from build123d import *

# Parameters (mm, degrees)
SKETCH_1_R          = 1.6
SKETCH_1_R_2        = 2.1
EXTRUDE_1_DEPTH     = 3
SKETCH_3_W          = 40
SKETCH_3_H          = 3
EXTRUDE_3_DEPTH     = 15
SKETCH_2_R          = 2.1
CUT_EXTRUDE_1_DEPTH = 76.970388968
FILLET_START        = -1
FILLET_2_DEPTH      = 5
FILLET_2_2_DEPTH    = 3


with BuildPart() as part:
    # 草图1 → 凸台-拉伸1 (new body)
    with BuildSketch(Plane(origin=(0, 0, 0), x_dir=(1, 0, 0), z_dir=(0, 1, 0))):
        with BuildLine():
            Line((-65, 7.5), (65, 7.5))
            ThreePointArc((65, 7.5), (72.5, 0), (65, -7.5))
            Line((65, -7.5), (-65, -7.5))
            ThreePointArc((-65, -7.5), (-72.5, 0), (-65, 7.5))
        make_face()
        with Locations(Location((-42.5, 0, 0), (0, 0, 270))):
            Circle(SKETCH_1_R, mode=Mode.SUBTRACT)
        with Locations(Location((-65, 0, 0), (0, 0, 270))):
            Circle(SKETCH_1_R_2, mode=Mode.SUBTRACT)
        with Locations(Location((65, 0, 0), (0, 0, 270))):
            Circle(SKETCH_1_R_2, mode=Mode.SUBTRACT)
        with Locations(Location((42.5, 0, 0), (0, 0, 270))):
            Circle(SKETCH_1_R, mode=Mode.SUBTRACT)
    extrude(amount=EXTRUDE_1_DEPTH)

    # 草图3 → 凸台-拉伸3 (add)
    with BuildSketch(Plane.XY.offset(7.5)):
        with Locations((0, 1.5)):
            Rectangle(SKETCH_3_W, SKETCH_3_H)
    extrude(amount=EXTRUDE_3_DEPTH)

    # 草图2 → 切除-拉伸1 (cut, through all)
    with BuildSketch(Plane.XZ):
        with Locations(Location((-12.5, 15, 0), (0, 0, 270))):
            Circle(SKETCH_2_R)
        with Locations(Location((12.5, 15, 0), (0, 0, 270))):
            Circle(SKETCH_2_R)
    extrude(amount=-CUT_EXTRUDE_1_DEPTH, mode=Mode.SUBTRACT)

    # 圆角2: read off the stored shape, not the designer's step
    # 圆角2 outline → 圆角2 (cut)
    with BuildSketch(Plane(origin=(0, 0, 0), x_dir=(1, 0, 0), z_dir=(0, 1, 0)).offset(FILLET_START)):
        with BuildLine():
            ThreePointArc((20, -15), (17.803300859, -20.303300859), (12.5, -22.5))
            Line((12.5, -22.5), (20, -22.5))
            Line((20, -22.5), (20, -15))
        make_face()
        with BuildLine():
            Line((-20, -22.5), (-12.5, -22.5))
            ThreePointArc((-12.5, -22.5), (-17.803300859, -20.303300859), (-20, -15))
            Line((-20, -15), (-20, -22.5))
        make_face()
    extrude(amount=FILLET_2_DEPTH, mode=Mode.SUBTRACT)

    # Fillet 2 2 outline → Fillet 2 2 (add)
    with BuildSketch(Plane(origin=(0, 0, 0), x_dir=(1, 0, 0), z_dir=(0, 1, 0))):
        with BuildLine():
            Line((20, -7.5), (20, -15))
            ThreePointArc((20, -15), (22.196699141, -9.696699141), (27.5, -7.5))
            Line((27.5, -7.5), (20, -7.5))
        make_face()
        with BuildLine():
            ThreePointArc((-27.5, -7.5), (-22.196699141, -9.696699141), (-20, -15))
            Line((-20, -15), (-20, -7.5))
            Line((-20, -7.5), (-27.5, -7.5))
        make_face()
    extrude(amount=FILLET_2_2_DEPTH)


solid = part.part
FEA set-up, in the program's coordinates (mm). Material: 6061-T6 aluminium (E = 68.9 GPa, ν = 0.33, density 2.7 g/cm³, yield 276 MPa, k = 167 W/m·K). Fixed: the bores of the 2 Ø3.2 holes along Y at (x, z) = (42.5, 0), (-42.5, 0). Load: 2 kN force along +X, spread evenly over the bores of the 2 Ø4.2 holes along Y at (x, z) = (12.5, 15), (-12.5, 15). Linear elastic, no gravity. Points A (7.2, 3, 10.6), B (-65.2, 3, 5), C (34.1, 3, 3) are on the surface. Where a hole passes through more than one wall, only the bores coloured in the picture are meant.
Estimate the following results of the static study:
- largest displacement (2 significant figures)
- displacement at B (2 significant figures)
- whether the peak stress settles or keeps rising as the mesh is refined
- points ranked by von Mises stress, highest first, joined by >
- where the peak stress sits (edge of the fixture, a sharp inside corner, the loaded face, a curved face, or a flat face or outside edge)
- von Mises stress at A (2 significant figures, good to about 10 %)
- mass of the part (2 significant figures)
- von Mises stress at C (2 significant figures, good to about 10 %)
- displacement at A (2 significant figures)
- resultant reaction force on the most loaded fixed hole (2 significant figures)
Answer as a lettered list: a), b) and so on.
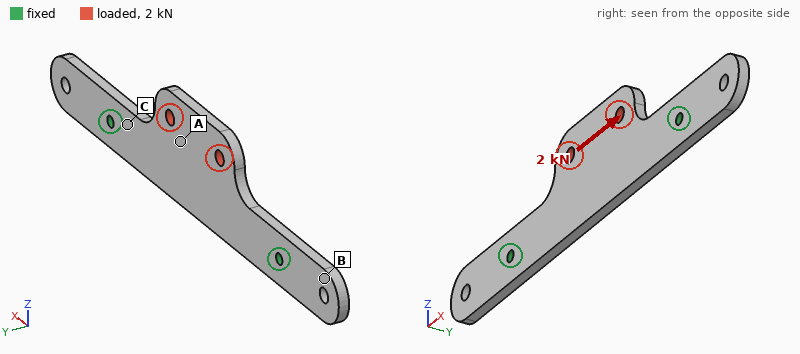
a) 30 µm
b) 11 µm
c) keeps rising
d) C > A > B
e) edge of the fixture
f) 21 MPa
g) 22 g
h) 39 MPa
i) 19 µm
j) 1.1 kN
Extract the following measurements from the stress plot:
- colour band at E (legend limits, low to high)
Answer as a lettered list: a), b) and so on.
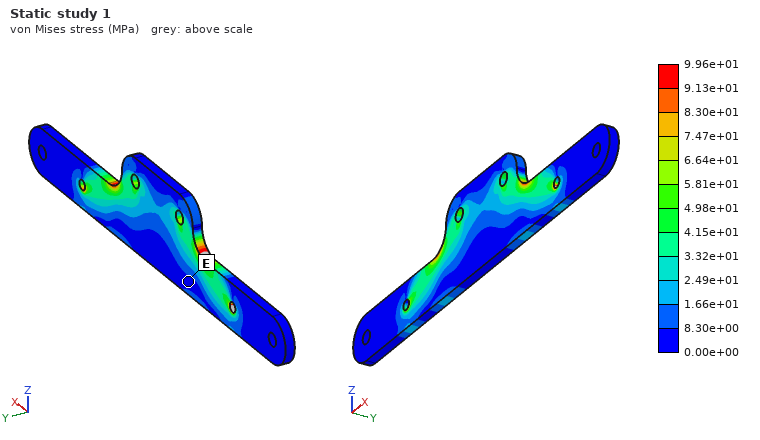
a) 0.00e+00 to 8.30e+00 MPa
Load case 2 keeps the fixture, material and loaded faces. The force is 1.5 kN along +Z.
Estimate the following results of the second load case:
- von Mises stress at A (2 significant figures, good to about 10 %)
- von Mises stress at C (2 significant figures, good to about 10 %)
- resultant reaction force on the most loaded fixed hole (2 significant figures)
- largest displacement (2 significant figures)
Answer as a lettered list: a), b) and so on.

a) 26 MPa
b) 41 MPa
c) 870 N
d) 73 µm
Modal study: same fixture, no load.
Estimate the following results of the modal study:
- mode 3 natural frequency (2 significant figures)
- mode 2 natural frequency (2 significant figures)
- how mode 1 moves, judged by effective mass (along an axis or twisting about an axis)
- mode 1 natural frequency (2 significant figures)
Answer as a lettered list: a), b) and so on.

a) 3100 Hz
b) 3100 Hz
c) along Y
d) 1600 Hz
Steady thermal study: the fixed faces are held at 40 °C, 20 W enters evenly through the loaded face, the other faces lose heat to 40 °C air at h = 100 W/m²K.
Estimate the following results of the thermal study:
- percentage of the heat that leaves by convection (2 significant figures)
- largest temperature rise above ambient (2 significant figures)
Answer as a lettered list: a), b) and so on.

a) 42 %
b) 34 K
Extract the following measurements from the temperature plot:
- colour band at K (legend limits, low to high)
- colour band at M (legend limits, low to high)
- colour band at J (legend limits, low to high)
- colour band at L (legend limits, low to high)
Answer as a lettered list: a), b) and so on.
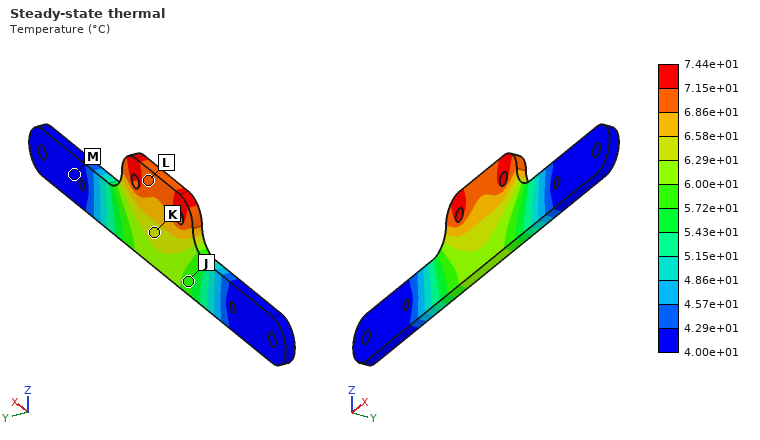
a) 6.29e+01 to 6.58e+01 °C
b) 4.00e+01 to 4.29e+01 °C
c) 5.72e+01 to 6.00e+01 °C
d) 6.86e+01 to 7.15e+01 °C
